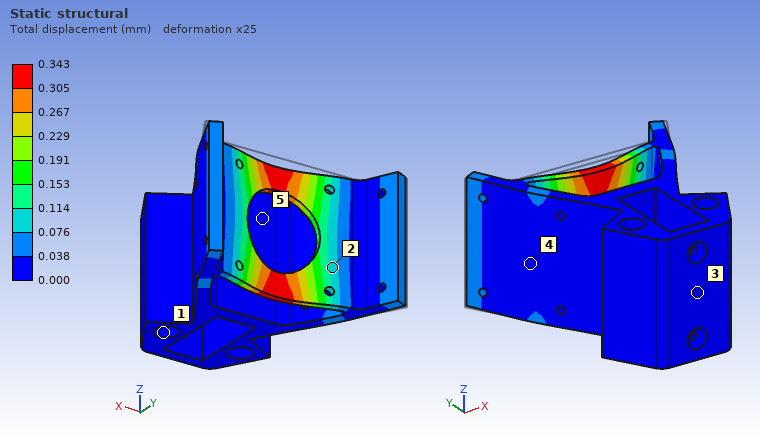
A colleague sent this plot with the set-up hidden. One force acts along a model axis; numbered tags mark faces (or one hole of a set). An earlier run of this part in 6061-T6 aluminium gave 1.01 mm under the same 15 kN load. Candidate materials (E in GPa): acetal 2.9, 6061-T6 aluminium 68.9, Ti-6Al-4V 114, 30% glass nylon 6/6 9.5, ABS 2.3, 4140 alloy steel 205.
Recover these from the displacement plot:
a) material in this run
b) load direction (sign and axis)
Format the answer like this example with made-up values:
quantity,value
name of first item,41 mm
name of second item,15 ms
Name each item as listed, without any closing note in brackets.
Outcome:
quantity,value
material in this run,4140 alloy steel
load direction,-Y
